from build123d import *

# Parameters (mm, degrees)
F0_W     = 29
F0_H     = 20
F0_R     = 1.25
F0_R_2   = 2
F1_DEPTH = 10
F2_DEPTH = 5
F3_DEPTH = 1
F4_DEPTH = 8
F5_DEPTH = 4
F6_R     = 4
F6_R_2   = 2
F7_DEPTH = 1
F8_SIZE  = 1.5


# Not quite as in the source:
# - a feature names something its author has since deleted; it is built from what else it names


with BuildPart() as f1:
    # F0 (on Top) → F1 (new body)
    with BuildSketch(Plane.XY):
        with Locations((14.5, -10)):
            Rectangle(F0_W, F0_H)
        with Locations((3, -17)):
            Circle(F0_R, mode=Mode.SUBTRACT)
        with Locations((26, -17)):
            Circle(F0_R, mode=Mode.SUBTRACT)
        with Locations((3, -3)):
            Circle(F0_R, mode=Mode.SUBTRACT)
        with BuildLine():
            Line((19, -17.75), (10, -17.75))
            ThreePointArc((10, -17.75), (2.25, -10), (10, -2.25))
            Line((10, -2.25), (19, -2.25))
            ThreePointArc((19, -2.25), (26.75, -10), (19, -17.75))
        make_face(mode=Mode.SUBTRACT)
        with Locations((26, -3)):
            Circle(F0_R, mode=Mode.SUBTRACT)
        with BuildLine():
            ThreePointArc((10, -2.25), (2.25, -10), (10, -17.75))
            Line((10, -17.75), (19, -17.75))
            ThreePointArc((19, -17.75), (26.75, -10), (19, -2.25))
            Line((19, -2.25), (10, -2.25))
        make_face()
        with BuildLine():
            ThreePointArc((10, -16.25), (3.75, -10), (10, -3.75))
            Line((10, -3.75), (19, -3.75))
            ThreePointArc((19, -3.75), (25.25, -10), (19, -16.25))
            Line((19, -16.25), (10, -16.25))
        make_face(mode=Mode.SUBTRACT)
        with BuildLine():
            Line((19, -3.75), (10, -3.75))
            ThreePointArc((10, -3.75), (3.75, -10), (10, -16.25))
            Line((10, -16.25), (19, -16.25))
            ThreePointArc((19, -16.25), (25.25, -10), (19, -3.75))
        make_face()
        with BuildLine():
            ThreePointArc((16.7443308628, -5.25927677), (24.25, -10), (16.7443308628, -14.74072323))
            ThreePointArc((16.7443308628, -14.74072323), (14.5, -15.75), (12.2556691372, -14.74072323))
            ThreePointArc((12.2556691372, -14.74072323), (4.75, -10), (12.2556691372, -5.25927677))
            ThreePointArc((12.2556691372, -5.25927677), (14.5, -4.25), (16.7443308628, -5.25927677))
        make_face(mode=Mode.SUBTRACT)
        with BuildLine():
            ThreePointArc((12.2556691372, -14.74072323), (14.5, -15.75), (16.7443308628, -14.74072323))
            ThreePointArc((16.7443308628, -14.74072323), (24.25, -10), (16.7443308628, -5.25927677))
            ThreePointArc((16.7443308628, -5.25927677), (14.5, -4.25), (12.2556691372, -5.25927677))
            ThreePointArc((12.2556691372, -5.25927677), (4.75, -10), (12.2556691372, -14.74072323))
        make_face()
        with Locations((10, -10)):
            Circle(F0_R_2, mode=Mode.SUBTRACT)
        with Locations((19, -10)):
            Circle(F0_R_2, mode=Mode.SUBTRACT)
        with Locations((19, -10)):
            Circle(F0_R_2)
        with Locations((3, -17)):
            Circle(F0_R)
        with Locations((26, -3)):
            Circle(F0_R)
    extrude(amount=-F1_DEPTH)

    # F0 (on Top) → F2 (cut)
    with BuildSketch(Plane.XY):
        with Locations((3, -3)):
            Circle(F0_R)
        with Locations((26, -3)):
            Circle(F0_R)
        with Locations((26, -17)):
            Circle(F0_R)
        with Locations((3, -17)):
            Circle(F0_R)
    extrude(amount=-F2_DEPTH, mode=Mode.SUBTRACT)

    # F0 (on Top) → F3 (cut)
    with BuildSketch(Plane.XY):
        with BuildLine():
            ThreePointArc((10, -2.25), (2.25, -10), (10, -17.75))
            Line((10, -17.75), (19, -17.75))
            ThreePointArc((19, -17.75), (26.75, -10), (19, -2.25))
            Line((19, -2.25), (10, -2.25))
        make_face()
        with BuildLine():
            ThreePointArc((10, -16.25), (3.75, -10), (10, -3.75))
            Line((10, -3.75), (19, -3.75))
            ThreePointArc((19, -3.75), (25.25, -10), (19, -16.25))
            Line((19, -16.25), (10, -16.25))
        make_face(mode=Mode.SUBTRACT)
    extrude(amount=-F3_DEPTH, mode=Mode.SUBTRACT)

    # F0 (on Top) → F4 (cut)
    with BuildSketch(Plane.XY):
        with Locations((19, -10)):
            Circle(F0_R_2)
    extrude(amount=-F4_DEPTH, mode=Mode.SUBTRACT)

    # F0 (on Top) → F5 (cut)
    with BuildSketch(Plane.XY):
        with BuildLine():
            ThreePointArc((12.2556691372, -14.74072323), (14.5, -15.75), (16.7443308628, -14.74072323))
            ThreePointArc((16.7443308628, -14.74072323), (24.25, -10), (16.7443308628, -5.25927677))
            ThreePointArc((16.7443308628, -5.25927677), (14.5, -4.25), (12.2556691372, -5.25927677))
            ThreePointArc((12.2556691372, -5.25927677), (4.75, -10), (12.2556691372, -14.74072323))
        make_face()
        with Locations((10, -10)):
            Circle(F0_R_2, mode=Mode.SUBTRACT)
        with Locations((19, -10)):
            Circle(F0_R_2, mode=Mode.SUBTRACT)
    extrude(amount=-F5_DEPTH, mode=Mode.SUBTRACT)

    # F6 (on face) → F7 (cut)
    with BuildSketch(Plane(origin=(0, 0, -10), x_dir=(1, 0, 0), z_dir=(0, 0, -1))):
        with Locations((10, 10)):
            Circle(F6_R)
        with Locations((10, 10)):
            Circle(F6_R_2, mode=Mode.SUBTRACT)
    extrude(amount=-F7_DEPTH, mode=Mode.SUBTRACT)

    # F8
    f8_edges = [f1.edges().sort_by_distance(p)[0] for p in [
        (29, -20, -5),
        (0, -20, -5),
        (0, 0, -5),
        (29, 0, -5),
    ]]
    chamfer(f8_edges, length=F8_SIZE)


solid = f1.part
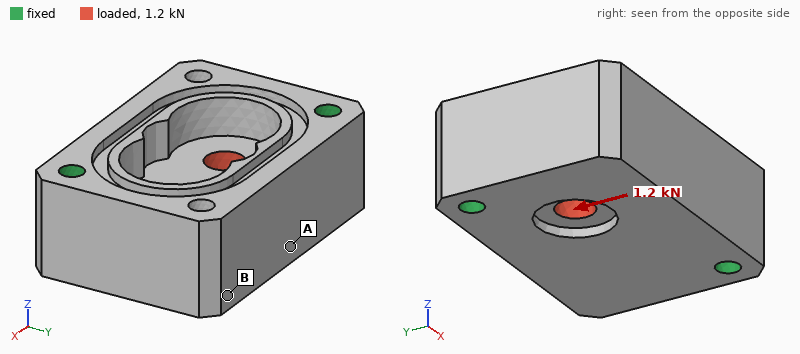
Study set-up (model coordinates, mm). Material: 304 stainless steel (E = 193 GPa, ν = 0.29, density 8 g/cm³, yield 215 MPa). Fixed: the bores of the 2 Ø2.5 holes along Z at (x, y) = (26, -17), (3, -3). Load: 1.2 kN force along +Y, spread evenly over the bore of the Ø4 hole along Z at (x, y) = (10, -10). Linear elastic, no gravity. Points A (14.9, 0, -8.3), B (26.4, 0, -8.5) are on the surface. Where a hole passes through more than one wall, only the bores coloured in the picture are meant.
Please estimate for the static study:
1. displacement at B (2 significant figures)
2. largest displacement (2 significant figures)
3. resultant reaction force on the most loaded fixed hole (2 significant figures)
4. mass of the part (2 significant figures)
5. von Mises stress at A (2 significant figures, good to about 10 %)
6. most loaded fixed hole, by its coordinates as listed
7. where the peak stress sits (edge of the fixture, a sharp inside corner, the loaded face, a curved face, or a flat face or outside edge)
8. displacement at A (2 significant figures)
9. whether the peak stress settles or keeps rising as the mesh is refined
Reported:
0.79 µm
1.3 µm
830 N
37 g
11 MPa
(3, -3)
edge of the fixture
0.96 µm
keeps rising
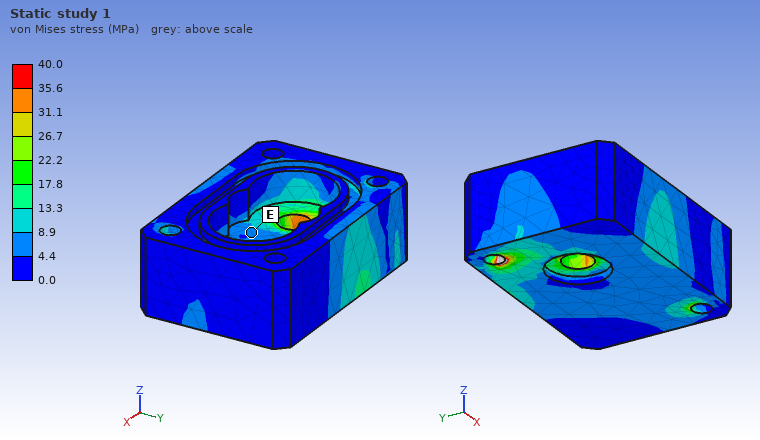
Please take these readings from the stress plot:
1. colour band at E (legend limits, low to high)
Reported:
4.4 to 8.9 MPa
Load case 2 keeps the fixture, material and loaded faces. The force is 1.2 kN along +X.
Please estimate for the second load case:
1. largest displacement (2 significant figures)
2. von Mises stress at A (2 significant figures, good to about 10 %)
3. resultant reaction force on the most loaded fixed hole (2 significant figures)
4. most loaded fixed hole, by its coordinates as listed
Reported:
1.1 µm
6.3 MPa
680 N
(3, -3)
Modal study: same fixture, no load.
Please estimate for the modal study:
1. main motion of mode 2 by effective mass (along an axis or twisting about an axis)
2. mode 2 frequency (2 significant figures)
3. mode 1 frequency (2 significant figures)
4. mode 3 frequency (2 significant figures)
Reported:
along Z
25 kHz
22 kHz
38 kHz
